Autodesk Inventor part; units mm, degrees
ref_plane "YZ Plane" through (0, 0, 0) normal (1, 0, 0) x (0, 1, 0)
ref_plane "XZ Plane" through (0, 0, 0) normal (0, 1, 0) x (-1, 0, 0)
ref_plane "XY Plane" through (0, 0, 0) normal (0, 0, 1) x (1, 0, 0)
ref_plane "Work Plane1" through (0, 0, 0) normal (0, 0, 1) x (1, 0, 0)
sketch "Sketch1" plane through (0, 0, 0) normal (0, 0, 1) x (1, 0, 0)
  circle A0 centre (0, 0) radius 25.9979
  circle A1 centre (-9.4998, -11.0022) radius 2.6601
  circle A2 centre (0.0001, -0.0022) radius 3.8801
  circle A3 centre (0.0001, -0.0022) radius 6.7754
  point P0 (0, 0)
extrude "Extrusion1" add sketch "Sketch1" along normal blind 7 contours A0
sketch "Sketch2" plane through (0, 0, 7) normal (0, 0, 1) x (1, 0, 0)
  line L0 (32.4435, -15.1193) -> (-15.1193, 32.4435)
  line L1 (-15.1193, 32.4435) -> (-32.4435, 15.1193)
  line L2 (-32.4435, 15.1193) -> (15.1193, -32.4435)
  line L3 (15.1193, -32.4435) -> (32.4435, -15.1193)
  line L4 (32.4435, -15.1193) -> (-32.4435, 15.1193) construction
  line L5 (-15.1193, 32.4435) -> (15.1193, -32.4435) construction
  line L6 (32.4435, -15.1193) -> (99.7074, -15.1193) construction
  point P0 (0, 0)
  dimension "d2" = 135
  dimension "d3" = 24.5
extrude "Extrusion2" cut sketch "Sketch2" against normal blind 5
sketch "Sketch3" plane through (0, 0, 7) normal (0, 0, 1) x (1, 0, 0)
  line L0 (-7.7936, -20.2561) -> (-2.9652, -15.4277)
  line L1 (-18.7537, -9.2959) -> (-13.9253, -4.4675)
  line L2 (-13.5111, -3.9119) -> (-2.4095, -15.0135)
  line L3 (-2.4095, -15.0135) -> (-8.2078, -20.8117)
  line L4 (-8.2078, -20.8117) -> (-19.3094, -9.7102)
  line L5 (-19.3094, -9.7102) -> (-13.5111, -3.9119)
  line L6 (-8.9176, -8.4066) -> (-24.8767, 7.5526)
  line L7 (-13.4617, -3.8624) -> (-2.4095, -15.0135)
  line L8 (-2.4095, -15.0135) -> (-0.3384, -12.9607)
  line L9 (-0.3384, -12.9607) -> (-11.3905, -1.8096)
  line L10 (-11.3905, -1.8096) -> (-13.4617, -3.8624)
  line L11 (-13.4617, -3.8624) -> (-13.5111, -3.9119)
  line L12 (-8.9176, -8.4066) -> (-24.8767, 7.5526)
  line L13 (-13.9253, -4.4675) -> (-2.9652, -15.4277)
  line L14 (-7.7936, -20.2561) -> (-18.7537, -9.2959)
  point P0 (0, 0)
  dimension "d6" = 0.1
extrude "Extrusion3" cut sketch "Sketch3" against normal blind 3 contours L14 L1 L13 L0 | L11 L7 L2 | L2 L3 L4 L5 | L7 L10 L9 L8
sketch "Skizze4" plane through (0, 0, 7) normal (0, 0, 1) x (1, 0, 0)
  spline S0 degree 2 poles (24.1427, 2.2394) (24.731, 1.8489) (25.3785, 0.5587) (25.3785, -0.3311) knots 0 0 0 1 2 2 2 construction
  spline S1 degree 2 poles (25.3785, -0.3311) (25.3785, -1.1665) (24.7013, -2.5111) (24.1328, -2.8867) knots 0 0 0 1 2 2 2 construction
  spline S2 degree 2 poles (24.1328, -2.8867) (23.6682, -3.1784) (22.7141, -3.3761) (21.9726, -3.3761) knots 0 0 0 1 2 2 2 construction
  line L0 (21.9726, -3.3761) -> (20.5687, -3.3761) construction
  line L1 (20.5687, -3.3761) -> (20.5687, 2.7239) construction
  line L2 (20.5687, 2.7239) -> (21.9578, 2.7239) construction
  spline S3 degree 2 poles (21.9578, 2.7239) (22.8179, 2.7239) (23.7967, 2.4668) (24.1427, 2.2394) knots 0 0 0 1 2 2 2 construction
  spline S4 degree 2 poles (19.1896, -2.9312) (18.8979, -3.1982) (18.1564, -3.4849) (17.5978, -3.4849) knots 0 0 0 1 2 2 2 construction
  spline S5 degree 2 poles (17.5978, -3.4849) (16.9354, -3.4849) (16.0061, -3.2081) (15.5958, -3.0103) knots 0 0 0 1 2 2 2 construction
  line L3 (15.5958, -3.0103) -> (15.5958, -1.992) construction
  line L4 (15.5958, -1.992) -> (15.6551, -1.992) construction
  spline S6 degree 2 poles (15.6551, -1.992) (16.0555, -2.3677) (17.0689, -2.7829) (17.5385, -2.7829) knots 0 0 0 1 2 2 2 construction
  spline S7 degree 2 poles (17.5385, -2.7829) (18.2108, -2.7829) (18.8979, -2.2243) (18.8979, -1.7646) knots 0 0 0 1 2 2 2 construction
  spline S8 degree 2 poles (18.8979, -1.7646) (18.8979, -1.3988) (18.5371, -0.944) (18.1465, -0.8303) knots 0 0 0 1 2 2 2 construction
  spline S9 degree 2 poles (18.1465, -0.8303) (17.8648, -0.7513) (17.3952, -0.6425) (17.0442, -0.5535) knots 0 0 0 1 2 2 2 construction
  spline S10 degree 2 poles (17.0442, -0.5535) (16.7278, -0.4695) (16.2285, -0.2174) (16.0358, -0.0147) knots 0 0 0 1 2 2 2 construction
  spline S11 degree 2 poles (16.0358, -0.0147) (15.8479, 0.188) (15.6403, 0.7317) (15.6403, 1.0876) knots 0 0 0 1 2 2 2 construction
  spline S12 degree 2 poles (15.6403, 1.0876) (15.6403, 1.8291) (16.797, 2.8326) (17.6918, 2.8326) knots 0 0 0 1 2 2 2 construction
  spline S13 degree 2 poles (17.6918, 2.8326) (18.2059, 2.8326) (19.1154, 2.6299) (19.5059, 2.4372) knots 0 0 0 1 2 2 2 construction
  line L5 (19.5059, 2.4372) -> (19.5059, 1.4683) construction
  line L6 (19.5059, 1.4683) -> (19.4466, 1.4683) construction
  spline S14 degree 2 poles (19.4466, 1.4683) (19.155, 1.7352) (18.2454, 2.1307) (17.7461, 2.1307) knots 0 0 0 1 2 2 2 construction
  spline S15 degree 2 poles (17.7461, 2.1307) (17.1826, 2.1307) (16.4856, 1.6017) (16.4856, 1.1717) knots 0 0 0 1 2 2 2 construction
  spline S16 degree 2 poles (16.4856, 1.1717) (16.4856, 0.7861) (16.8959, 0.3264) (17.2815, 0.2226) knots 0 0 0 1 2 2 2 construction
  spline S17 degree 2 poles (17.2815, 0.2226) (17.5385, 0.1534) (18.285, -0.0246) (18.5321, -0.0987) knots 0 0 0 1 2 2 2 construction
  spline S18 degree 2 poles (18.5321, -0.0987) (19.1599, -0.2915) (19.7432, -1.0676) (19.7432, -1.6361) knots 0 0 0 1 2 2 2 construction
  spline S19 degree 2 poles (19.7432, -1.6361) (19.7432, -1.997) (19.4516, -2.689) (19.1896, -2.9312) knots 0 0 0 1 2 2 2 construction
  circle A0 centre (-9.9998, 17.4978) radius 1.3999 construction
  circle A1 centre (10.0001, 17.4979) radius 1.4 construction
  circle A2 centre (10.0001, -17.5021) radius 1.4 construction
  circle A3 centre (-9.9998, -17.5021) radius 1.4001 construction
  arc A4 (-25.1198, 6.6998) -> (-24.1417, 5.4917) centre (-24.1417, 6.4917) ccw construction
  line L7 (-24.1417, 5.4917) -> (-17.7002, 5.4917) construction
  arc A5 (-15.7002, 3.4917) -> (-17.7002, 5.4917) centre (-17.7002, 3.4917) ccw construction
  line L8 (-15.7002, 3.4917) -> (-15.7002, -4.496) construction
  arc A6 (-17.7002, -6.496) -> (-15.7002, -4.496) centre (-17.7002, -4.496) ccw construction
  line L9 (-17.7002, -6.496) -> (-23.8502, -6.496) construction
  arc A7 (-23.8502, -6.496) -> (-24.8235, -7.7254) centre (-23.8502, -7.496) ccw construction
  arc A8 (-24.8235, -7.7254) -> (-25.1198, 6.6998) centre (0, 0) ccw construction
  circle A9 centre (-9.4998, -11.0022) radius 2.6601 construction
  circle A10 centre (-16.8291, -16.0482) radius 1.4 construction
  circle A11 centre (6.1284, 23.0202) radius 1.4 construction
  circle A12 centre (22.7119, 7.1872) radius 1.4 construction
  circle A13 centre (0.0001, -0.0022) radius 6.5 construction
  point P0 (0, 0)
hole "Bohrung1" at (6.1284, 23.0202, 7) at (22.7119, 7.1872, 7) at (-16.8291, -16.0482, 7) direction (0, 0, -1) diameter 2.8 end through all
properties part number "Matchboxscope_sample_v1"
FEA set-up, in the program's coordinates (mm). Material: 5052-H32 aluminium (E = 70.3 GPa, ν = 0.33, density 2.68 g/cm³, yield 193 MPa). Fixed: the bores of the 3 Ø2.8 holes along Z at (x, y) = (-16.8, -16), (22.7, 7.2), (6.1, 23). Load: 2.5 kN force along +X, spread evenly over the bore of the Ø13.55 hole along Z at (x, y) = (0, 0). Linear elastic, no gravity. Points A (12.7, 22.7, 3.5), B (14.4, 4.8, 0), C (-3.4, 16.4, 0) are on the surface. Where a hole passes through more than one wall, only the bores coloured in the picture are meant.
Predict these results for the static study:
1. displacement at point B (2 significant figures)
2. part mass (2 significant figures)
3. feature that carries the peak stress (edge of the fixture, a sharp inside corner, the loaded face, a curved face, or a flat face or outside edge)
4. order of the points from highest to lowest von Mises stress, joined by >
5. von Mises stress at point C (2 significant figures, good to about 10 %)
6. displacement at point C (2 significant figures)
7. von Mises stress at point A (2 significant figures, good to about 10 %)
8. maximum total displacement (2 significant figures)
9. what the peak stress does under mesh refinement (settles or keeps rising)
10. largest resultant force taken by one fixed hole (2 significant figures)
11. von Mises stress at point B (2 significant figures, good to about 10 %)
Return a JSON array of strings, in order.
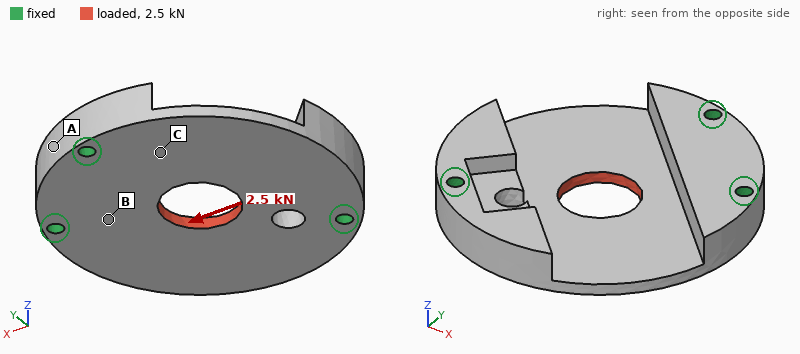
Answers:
["4.2 µm", "21 g", "edge of the fixture", "B > C > A", "17 MPa", "6.0 µm", "7.8 MPa", "17 µm", "keeps rising", "1.0 kN", "33 MPa"]
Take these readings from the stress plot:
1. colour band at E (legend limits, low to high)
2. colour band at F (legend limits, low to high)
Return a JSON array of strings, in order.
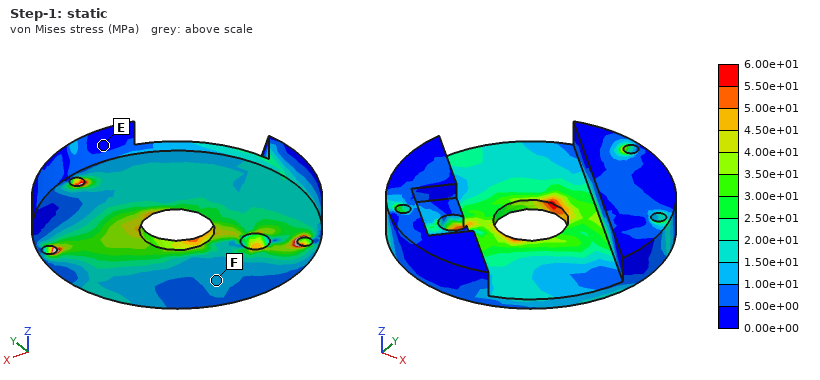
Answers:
["0.00e+00 to 5.00e+00 MPa", "1.00e+01 to 1.50e+01 MPa"]
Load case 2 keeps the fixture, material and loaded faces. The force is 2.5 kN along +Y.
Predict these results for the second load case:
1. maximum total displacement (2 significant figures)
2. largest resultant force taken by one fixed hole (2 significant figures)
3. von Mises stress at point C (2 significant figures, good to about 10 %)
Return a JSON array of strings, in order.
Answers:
["19 µm", "1.0 kN", "22 MPa"]
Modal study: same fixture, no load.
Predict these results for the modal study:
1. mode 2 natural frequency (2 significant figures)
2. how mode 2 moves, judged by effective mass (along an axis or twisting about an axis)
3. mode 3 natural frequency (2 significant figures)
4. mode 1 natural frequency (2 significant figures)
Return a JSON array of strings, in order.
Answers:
["8200 Hz", "along Z", "14 kHz", "7400 Hz"]
